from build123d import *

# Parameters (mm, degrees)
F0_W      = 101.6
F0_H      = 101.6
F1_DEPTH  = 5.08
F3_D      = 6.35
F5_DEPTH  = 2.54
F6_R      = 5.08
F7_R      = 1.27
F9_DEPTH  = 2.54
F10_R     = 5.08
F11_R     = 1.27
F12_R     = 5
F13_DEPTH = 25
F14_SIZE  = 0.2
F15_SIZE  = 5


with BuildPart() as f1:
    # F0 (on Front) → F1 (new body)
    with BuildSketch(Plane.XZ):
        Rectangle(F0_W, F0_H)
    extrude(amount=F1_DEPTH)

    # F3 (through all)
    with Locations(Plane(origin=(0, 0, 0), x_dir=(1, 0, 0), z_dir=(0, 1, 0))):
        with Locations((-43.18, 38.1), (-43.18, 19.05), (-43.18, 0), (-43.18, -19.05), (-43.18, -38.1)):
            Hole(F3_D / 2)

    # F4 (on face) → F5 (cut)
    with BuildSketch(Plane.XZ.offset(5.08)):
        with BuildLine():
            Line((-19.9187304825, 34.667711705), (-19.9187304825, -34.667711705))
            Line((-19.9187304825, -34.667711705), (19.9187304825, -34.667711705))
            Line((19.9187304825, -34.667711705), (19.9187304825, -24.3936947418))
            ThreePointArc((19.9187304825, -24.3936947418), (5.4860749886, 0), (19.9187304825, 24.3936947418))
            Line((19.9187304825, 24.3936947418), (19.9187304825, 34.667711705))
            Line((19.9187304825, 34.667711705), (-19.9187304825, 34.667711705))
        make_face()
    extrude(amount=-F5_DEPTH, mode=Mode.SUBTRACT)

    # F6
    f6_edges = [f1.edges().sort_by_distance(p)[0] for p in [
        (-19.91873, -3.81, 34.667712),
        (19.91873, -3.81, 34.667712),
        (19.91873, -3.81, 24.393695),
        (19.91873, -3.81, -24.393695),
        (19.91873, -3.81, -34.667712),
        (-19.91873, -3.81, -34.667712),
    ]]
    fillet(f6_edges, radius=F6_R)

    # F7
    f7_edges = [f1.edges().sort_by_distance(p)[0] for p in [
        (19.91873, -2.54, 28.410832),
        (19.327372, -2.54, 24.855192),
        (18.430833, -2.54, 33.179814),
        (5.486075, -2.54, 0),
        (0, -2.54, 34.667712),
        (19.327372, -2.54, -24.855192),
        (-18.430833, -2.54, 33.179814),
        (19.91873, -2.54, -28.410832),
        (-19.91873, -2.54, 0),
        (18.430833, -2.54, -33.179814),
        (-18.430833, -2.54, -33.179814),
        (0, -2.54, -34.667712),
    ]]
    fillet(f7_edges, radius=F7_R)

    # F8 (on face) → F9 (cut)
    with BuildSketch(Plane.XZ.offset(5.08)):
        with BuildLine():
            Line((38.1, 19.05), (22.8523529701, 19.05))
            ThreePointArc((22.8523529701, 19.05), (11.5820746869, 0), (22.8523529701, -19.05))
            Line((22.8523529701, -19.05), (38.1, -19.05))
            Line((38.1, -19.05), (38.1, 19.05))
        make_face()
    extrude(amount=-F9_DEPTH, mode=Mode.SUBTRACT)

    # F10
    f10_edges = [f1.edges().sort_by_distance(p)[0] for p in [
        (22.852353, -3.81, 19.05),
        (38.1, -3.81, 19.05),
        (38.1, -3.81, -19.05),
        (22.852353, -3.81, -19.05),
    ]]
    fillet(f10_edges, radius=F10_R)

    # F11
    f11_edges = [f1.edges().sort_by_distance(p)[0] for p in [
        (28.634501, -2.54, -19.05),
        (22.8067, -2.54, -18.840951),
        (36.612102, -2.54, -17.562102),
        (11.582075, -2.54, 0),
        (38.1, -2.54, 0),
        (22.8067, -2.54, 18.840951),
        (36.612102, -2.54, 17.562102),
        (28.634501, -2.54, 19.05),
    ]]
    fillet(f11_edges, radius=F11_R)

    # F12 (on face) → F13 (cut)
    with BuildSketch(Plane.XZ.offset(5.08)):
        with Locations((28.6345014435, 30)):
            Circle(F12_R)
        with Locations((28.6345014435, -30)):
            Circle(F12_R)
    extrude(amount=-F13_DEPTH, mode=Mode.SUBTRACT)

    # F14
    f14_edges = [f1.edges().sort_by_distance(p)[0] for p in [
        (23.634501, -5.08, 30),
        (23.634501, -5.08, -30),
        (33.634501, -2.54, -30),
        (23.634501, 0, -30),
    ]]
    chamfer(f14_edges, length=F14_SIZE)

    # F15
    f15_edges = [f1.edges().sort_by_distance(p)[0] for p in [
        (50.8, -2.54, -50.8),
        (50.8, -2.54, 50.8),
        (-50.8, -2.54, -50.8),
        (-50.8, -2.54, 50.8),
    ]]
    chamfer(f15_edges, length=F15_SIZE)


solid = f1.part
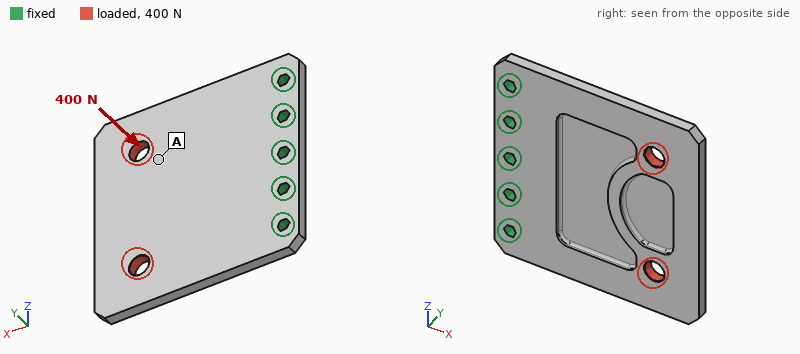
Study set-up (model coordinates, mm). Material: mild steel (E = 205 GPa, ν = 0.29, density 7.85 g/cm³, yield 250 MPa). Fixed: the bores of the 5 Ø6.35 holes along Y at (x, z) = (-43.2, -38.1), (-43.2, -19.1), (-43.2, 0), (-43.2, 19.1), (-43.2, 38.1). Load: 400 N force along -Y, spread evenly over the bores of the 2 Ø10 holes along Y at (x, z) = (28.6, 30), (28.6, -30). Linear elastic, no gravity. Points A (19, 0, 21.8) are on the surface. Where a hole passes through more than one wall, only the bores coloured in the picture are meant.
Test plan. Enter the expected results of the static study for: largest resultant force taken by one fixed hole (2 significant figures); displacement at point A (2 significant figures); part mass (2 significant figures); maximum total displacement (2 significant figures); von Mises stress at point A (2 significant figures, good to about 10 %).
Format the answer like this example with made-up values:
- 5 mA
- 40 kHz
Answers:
- 530 N
- 0.23 mm
- 340 g
- 0.45 mm
- 11 MPa
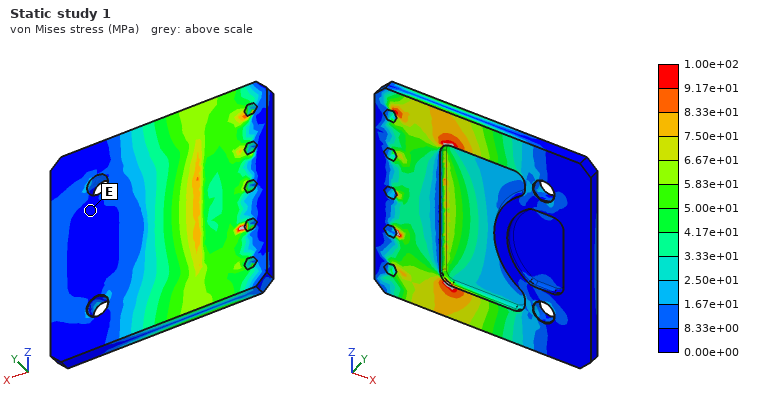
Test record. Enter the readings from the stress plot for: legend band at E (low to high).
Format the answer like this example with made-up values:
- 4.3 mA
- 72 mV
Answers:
- 0.00e+00 to 8.33e+00 MPa
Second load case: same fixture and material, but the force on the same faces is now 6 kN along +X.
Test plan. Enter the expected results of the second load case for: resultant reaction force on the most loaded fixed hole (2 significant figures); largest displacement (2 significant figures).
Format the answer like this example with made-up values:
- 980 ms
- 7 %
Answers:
- 1.8 kN
- 89 µm
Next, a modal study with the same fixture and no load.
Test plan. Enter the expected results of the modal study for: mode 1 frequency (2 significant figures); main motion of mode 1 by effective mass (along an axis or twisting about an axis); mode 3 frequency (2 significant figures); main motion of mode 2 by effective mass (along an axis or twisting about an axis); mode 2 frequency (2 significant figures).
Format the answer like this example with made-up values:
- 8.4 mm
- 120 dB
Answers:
- 440 Hz
- along Y
- 2500 Hz
- twisting about X
- 940 Hz
